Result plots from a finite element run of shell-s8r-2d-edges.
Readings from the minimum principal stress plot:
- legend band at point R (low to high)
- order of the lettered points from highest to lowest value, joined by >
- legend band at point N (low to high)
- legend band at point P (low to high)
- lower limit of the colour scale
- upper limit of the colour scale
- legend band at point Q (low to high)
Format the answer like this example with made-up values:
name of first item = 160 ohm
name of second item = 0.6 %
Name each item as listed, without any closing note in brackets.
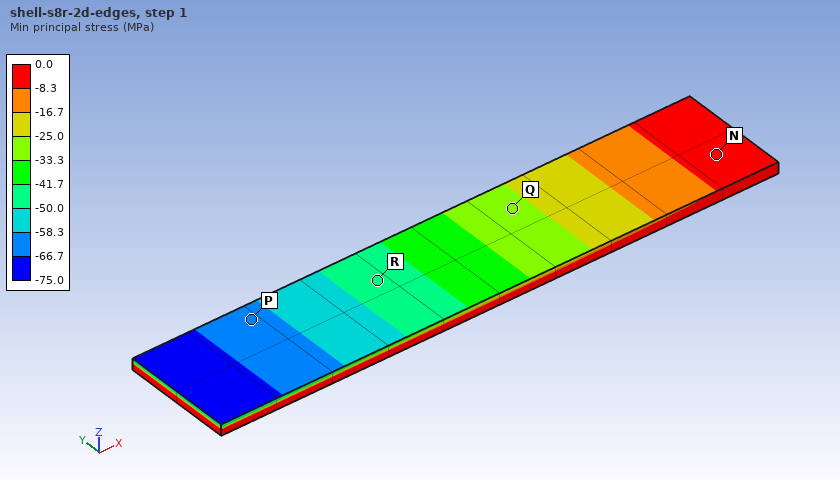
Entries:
legend band at point R = -50.0 to -41.7 MPa
order of the lettered points from highest to lowest value, joined by > = N > Q > R > P
legend band at point N = -8.3 to 0.0 MPa
legend band at point P = -66.7 to -58.3 MPa
lower limit of the colour scale = -75.0 MPa
upper limit of the colour scale = 0.0 MPa
legend band at point Q = -33.3 to -25.0 MPa
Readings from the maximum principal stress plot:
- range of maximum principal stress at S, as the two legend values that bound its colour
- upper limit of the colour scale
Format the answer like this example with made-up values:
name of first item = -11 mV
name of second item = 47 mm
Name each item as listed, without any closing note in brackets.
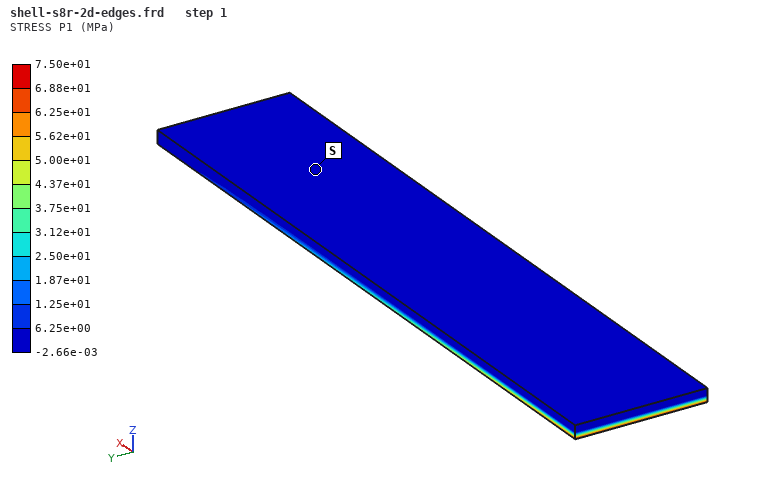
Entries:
range of maximum principal stress at S, as the two legend values that bound its colour = -2.66e-03 to 6.25e+00 MPa
upper limit of the colour scale = 7.50e+01 MPa
